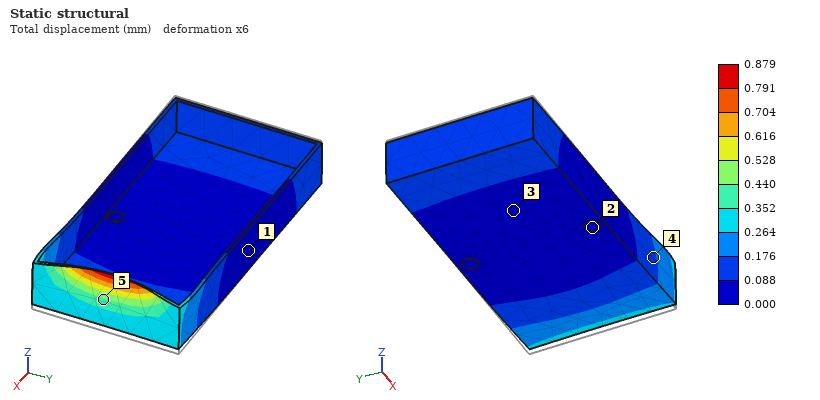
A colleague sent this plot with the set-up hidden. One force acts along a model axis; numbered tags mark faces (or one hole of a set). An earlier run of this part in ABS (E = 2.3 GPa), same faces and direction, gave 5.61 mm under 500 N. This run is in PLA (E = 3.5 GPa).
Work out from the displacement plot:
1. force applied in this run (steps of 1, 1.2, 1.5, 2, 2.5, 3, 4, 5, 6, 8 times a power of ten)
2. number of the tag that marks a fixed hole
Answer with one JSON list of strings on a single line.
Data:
["120 N", "2"]
